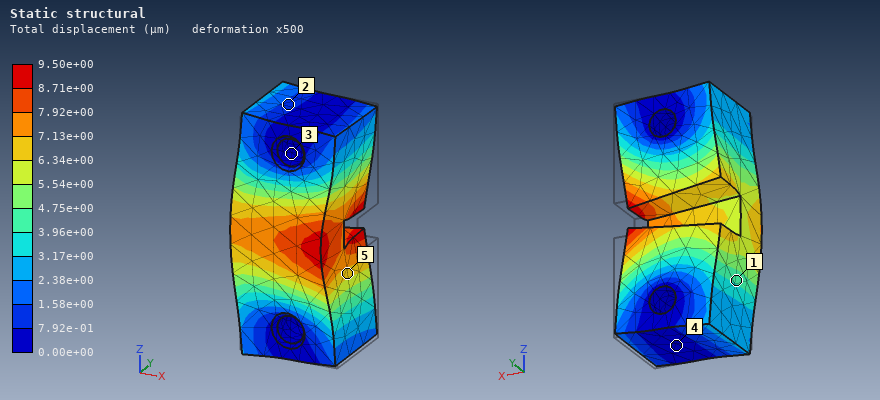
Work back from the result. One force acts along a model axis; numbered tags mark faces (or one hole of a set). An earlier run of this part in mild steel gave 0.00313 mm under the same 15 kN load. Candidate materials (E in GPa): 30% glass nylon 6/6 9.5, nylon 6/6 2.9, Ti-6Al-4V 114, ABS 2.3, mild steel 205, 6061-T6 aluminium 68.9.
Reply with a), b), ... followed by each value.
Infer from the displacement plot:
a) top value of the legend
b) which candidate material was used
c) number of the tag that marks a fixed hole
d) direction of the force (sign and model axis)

a) 9.50e+00 µm
b) 6061-T6 aluminium
c) 3
d) -X
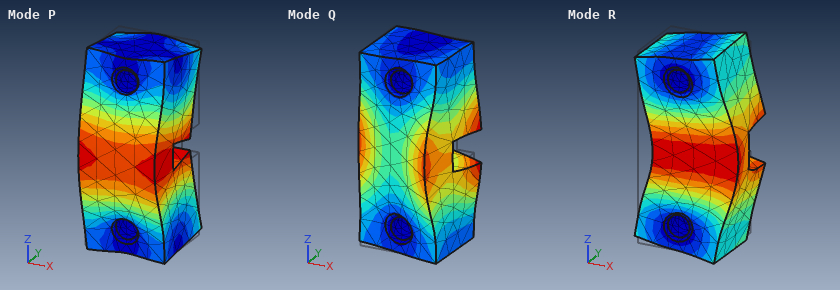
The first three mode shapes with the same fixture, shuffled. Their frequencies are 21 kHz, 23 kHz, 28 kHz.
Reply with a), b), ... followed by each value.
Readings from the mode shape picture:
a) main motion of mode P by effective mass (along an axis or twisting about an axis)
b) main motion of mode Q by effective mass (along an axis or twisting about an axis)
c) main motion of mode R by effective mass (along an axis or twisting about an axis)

a) along Y
b) twisting about Z
c) along X
